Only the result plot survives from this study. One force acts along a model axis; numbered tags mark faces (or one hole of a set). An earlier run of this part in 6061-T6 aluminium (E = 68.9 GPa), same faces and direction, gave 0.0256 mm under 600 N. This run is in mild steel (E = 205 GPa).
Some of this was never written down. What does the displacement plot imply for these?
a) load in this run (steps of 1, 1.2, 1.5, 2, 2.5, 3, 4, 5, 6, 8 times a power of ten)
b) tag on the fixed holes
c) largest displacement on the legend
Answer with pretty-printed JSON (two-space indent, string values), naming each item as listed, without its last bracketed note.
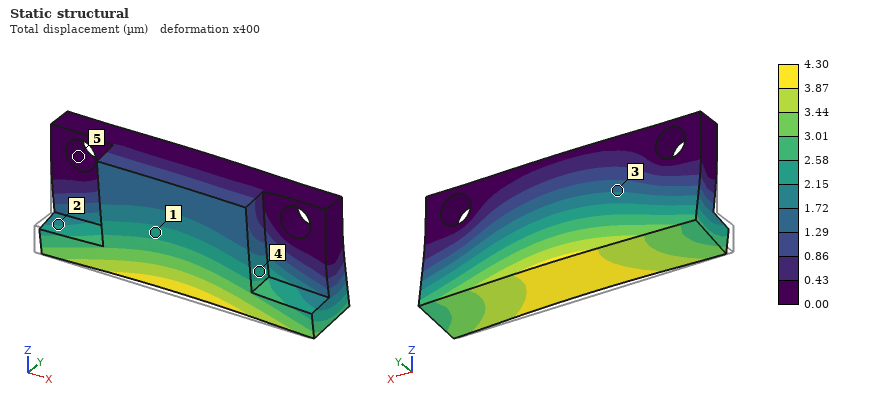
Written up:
{
  "load in this run": "300 N",
  "tag on the fixed holes": "5",
  "largest displacement on the legend": "4.30 µm"
}
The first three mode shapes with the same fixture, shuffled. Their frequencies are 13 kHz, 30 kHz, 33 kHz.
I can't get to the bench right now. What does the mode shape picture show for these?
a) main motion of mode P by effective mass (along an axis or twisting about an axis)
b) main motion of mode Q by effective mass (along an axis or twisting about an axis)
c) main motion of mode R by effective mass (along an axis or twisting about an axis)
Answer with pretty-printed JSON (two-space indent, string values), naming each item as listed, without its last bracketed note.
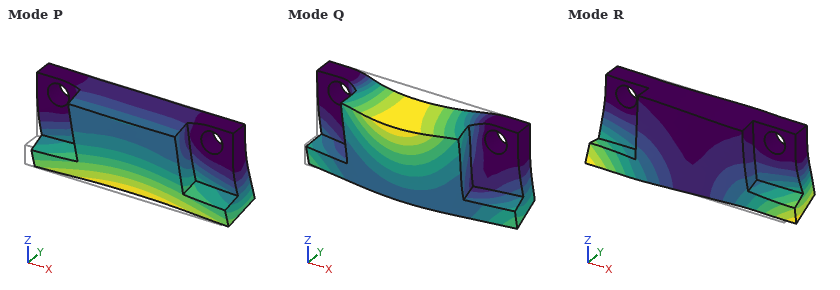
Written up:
{
  "main motion of mode P by effective mass": "along Y",
  "main motion of mode Q by effective mass": "along Y",
  "main motion of mode R by effective mass": "twisting about Z"
}
